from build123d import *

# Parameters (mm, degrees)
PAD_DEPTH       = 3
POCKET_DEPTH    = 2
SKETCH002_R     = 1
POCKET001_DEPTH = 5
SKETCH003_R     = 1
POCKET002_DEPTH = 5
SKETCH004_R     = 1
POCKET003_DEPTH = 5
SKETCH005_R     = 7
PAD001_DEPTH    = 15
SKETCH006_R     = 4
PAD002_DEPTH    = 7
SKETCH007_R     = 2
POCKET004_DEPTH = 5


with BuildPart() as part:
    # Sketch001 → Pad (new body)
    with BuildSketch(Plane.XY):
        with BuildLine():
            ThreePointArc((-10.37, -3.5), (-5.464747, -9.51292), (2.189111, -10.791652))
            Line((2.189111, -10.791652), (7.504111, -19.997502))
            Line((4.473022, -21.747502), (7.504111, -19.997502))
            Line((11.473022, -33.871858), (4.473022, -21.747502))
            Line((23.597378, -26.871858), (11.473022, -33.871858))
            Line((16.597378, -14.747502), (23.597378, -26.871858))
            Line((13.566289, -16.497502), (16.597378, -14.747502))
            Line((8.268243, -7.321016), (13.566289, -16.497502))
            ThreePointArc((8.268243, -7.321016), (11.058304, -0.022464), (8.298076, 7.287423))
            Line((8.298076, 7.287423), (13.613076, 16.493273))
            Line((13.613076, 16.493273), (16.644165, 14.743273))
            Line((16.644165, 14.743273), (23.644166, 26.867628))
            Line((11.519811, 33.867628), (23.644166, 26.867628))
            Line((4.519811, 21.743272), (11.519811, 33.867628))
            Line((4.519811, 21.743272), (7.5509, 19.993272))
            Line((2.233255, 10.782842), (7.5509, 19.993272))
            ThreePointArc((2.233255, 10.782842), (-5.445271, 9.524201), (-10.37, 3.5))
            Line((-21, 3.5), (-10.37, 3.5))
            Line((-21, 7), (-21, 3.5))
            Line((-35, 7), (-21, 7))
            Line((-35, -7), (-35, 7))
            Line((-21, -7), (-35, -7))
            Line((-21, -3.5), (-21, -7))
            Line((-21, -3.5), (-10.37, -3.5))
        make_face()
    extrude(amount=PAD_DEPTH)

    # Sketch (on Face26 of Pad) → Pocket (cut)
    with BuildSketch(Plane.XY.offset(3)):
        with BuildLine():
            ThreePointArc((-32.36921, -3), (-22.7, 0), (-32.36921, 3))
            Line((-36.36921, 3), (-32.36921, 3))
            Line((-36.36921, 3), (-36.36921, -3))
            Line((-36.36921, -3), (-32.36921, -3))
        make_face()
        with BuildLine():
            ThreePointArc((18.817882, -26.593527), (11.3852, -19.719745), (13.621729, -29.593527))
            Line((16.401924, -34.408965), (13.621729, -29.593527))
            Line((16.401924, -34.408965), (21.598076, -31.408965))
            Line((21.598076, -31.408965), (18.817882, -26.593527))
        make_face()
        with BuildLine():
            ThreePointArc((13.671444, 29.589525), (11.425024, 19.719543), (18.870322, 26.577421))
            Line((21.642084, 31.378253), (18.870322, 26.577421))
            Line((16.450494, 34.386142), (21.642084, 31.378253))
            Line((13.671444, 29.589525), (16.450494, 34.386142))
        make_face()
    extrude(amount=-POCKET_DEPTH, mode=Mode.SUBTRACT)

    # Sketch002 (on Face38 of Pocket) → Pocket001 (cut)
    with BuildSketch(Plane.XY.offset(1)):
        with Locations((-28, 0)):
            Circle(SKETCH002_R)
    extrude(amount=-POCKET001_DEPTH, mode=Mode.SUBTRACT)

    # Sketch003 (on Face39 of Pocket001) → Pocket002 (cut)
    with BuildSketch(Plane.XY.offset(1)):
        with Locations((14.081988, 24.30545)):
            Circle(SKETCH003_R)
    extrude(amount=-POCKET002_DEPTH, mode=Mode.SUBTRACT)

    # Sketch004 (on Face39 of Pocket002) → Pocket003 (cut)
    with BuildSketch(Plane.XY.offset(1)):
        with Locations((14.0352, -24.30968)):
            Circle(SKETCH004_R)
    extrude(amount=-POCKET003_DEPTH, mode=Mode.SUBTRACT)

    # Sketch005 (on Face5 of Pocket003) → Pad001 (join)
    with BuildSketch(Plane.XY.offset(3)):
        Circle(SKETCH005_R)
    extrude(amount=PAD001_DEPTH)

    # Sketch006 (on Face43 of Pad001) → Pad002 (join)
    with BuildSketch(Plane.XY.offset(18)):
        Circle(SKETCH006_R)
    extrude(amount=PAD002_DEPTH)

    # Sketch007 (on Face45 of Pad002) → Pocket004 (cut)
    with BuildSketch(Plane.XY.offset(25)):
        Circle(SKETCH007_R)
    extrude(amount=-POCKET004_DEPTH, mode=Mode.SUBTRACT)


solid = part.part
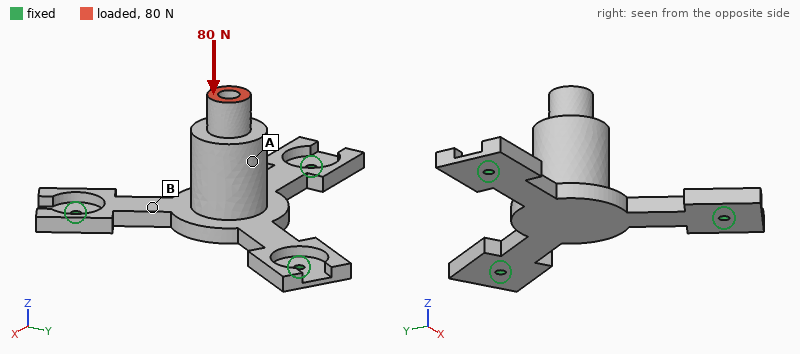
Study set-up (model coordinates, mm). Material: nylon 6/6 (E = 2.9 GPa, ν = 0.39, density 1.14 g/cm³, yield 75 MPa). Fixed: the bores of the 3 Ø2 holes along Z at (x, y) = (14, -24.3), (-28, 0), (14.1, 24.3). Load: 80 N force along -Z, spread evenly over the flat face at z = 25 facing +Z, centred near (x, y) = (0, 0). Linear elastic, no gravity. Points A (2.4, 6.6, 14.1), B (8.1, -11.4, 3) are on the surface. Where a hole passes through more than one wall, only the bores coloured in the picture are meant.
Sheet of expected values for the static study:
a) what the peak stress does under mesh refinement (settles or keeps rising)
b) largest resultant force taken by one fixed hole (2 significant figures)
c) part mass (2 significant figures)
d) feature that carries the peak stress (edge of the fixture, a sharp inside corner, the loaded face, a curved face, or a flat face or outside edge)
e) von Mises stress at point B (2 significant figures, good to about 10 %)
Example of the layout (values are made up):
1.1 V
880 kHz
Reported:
keeps rising
97 N
6.3 g
edge of the fixture
19 MPa
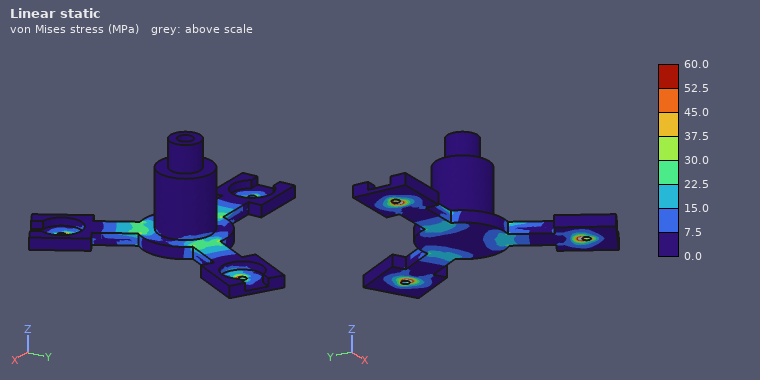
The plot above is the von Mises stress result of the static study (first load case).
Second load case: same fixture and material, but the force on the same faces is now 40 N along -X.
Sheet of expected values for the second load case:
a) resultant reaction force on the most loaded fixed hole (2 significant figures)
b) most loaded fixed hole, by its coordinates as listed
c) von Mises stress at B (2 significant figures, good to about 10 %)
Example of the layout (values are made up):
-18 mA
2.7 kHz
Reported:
40 N
(-28, 0)
13 MPa
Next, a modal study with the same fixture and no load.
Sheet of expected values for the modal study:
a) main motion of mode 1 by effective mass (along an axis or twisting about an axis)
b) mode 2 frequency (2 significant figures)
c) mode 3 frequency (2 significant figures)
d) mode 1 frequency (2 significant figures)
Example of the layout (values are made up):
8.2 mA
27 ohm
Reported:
along Z
1100 Hz
1100 Hz
710 Hz
